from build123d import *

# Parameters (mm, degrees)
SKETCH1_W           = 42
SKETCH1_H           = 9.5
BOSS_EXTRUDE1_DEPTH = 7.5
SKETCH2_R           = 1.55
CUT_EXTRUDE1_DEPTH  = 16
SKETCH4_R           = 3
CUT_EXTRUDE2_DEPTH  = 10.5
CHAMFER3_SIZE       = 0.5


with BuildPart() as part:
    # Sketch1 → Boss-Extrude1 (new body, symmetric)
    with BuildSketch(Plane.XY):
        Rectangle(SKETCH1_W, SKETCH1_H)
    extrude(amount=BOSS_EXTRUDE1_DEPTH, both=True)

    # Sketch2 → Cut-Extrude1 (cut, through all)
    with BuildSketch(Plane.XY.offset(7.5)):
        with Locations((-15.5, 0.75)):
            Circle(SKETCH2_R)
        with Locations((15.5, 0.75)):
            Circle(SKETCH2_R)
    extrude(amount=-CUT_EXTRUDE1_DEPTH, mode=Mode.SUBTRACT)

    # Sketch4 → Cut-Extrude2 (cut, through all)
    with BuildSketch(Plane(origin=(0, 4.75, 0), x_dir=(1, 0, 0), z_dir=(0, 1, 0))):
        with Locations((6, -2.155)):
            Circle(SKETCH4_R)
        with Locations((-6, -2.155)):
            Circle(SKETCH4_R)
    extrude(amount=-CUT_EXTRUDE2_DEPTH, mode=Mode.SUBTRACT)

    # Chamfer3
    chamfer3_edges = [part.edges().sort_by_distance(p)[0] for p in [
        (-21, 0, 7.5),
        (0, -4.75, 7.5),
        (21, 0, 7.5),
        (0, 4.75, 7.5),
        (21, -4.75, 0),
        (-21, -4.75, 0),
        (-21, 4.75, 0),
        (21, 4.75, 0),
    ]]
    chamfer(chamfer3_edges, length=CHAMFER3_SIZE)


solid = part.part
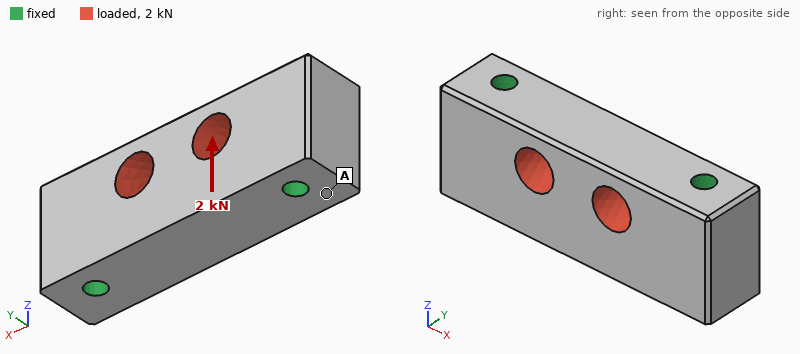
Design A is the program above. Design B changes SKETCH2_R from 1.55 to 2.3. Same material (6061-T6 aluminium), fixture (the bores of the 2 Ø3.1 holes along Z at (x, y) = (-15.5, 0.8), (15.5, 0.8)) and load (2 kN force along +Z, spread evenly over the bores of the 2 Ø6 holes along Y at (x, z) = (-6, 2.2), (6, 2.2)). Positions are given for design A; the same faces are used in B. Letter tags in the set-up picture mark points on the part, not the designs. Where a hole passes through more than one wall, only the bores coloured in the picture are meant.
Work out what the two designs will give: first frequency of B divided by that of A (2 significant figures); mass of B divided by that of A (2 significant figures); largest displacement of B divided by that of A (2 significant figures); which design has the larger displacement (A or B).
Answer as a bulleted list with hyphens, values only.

- 1.2
- 0.95
- 0.90
- A
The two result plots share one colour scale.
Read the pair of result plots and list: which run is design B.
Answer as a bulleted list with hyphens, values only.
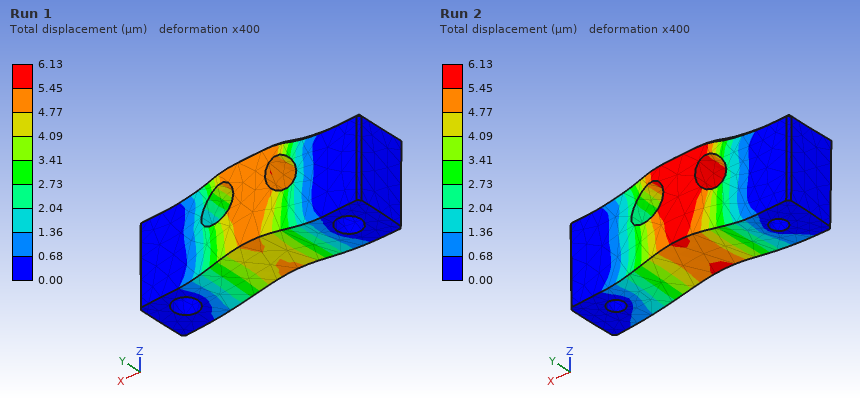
- Run 1
